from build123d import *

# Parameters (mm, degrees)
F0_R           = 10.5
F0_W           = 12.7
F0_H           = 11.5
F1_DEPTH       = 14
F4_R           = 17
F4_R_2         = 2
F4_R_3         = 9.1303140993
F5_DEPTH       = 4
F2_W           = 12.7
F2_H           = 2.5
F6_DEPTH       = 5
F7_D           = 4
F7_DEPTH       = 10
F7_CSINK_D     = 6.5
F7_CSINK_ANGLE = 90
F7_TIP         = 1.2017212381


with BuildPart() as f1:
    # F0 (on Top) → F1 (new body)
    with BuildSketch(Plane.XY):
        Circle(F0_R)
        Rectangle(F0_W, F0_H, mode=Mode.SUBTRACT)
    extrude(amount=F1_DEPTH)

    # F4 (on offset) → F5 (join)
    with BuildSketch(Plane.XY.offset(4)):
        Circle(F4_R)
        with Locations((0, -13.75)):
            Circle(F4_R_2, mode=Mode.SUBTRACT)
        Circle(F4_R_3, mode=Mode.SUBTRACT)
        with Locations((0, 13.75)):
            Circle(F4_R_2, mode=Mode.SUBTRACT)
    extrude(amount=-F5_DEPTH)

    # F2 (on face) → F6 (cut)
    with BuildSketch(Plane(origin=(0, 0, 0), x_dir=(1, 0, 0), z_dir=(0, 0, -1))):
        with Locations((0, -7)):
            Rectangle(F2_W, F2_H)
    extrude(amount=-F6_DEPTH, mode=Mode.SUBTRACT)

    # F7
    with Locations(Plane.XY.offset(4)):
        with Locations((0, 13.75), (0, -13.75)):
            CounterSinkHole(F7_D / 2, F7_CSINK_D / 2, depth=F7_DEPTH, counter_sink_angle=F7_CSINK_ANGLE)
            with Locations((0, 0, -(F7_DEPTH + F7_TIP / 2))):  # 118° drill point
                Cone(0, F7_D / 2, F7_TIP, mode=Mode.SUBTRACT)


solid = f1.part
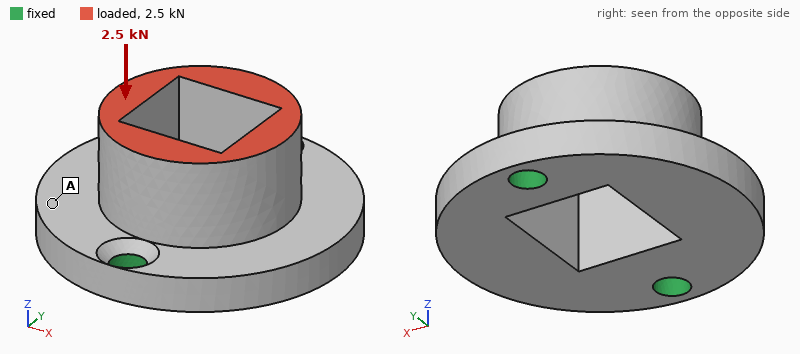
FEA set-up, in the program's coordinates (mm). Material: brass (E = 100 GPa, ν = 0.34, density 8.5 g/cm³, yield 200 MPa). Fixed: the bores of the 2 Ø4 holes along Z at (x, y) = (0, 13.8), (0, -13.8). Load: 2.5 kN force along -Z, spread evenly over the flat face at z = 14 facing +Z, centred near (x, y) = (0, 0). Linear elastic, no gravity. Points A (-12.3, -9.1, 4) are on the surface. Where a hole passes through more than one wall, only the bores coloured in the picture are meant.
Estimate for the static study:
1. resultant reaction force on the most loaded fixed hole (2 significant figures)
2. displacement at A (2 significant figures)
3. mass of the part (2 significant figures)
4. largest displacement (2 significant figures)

1.4 kN
10 µm
41 g
15 µm
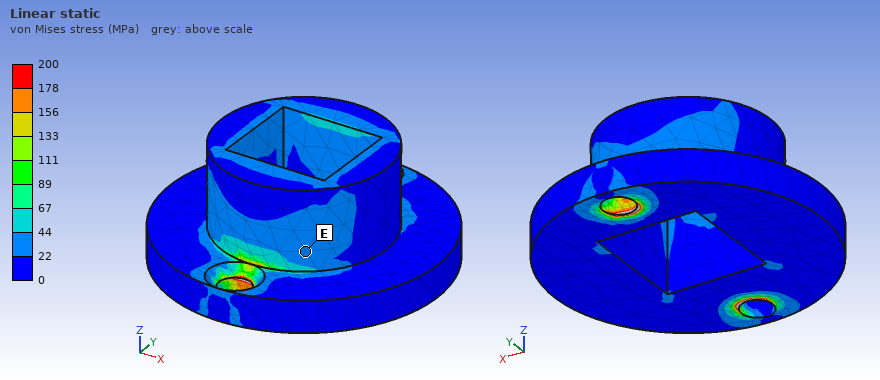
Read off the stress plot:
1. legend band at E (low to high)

22 to 44 MPa
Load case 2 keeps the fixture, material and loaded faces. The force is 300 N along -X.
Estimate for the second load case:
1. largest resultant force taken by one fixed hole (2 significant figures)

150 N
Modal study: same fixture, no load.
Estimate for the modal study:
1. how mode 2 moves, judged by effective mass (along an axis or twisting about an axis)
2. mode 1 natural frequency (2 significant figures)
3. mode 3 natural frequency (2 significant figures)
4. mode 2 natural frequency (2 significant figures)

along Z
5000 Hz
17 kHz
11 kHz
